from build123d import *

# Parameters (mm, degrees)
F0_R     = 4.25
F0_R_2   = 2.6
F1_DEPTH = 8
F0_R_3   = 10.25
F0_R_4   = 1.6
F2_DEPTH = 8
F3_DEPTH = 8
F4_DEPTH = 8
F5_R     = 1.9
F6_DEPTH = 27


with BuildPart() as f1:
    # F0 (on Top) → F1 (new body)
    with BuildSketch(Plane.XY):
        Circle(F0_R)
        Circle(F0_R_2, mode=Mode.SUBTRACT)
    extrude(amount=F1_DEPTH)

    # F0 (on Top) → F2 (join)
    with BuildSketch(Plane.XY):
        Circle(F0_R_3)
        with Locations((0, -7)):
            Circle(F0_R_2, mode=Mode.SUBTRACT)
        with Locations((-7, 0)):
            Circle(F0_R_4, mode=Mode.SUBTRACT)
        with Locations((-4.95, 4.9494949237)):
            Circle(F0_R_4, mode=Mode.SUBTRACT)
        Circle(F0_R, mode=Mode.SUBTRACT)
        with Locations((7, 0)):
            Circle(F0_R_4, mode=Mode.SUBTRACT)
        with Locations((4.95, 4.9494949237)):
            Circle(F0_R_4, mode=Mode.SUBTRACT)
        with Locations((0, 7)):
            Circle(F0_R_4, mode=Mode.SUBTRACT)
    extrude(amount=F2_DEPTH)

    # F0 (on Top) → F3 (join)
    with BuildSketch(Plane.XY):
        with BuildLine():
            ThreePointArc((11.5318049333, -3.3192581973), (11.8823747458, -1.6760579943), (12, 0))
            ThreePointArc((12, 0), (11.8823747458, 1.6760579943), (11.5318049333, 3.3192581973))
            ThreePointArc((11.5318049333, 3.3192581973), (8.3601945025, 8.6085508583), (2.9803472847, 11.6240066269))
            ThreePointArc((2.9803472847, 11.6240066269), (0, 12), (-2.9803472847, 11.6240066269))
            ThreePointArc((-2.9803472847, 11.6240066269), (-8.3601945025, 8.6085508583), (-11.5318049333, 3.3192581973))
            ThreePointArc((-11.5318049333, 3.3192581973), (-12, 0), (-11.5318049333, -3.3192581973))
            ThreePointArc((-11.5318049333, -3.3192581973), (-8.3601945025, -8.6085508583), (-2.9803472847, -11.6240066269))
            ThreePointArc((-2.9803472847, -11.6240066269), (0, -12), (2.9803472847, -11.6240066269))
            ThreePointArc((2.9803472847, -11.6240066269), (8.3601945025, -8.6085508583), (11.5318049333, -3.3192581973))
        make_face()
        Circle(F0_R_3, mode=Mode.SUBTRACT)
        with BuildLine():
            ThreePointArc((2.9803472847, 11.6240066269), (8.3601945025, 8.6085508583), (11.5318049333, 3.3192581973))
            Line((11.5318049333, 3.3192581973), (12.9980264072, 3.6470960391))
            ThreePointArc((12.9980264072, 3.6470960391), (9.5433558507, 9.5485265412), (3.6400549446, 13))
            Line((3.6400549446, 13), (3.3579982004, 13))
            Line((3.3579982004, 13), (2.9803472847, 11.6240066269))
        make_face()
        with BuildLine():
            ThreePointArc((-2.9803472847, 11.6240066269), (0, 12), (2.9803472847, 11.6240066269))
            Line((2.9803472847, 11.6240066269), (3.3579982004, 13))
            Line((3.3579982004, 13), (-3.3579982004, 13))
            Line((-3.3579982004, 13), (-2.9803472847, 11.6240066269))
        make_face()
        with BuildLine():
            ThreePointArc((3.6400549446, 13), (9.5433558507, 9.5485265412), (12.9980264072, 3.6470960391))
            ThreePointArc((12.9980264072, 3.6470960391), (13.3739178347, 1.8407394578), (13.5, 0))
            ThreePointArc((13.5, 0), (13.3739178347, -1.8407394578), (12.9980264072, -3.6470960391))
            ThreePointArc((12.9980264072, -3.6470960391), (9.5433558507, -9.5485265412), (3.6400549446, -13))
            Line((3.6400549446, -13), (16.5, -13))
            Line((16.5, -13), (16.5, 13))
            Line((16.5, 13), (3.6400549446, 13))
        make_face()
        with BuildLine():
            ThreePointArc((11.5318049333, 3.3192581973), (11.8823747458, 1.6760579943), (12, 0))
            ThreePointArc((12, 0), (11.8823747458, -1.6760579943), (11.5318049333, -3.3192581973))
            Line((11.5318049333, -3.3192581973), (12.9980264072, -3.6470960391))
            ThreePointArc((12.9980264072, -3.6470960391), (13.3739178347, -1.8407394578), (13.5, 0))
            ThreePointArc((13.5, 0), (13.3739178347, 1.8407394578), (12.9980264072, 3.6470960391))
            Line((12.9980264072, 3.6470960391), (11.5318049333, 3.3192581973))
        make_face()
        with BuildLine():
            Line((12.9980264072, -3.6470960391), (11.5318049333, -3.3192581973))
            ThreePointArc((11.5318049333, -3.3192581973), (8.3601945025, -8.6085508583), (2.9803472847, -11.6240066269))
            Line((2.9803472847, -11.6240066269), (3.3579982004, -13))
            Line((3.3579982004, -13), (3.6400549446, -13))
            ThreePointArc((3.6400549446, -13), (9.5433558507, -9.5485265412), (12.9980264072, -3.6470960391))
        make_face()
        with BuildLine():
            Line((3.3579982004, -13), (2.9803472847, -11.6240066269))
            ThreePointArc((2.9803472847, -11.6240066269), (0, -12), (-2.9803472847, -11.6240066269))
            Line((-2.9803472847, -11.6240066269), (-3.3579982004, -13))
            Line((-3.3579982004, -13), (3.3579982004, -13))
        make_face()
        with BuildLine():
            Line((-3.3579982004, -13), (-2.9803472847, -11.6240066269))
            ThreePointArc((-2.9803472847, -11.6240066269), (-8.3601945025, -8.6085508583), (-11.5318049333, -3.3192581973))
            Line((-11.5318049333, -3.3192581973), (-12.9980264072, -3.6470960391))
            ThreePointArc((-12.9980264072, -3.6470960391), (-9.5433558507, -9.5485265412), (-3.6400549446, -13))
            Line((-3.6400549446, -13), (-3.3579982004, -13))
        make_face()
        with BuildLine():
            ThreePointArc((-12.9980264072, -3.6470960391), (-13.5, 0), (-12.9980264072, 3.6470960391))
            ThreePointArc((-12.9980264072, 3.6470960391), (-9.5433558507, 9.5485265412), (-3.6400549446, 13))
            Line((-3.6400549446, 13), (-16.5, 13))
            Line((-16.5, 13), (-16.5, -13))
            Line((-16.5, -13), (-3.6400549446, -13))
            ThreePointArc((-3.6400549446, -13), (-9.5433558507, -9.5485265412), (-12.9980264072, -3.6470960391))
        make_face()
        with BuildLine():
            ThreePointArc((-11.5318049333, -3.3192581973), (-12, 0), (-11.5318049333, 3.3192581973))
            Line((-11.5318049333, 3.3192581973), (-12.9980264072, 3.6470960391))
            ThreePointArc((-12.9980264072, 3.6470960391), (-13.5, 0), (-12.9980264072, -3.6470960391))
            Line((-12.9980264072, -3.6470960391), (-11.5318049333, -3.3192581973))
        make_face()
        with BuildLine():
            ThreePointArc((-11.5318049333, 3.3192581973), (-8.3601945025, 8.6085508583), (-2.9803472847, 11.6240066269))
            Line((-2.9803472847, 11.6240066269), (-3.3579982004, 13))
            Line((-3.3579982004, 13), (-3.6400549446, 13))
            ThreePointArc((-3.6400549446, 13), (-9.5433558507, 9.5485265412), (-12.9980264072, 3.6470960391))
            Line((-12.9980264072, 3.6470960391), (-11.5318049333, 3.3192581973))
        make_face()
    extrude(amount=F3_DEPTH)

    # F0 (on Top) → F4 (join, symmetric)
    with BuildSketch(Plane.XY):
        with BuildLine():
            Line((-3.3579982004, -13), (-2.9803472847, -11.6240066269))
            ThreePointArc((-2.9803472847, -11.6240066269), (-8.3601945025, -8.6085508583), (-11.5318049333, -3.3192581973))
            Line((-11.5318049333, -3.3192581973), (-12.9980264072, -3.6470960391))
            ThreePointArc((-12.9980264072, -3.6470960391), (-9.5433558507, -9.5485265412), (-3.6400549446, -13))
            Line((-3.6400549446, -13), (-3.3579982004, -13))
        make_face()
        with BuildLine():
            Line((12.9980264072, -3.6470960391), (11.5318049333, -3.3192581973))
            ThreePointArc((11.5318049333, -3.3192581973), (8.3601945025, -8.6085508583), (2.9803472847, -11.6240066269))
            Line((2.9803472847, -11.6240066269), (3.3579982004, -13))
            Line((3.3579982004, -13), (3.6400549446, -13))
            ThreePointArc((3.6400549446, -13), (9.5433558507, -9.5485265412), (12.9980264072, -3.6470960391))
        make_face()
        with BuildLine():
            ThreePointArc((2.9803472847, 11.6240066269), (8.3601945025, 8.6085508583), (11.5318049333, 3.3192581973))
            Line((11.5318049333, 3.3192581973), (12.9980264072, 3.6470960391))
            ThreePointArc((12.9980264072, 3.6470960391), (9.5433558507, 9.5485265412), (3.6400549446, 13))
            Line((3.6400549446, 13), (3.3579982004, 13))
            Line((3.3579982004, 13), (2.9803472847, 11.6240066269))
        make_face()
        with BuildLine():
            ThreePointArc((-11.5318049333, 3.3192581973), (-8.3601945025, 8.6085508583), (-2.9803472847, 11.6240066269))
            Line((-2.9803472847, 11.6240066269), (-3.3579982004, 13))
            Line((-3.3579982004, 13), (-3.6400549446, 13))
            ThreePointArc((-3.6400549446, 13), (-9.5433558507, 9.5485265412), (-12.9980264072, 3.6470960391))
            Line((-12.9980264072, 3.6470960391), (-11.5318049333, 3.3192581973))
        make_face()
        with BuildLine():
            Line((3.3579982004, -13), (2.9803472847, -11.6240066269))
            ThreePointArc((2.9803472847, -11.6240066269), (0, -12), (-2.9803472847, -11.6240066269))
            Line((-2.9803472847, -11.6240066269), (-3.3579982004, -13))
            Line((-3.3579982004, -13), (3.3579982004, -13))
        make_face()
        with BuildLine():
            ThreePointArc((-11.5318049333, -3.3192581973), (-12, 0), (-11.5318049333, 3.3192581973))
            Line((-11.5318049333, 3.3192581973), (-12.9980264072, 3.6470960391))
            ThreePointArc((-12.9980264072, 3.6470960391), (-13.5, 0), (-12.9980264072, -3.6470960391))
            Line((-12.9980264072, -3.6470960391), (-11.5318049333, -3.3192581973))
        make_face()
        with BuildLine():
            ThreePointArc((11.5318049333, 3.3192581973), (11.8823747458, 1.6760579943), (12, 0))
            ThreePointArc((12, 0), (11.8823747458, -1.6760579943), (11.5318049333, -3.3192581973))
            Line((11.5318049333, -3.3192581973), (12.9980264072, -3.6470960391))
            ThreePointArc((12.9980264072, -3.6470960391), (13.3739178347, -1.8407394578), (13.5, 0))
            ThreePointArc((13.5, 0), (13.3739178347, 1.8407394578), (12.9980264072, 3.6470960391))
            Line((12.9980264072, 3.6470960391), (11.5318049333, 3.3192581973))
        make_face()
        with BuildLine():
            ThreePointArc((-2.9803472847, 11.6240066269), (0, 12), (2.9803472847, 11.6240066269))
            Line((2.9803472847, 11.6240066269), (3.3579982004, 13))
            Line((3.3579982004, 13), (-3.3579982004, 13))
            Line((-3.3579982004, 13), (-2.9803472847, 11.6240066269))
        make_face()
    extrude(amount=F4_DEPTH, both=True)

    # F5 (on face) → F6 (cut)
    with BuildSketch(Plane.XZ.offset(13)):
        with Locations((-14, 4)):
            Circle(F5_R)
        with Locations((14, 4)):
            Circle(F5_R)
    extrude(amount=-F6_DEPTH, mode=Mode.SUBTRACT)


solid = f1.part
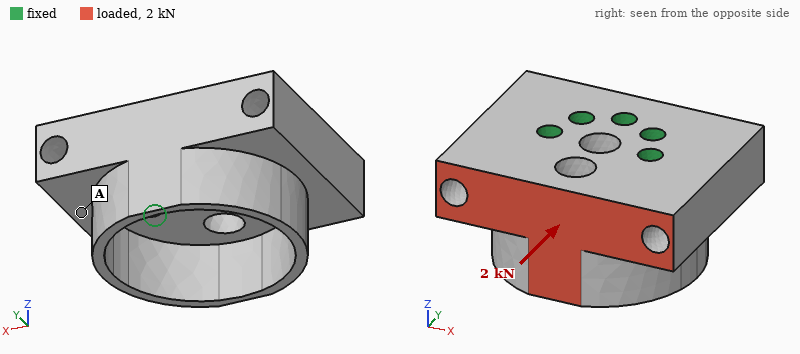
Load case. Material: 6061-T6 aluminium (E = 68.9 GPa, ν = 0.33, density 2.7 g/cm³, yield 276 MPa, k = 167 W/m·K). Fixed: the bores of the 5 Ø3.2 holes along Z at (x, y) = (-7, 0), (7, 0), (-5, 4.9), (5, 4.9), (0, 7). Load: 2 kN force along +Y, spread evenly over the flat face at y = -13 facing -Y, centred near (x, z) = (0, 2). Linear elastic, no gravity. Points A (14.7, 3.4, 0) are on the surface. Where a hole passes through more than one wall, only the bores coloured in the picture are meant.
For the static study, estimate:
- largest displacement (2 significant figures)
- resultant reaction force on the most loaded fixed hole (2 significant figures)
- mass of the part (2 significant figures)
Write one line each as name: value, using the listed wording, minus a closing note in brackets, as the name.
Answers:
largest displacement: 47 µm
resultant reaction force on the most loaded fixed hole: 870 N
mass of the part: 18 g
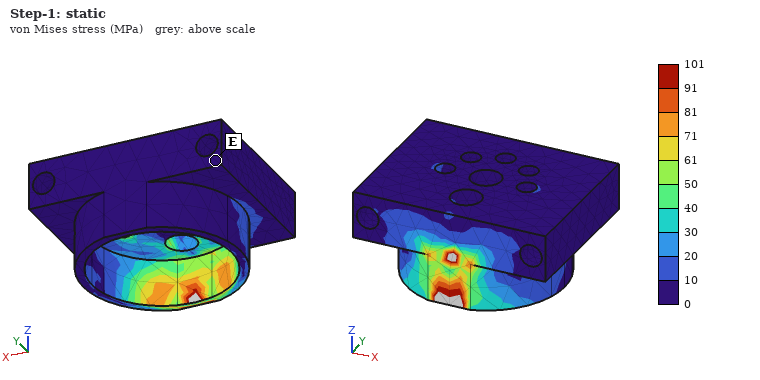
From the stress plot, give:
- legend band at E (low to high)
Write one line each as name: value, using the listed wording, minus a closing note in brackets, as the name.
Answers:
legend band at E: 0 to 10 MPa
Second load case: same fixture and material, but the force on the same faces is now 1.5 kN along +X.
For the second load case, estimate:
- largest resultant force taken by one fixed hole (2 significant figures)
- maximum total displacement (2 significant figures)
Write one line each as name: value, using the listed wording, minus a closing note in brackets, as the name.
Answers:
largest resultant force taken by one fixed hole: 1.3 kN
maximum total displacement: 13 µm
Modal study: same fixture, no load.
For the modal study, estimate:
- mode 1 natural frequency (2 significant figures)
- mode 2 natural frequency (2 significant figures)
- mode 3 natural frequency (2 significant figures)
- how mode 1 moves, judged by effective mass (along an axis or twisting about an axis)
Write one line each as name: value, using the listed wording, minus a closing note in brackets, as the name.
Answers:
mode 1 natural frequency: 24 kHz
mode 2 natural frequency: 25 kHz
mode 3 natural frequency: 30 kHz
how mode 1 moves, judged by effective mass: along Z
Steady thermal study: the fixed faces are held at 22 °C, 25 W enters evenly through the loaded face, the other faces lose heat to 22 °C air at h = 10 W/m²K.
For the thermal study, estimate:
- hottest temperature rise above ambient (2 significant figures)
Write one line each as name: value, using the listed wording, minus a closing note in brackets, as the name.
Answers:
hottest temperature rise above ambient: 15 K
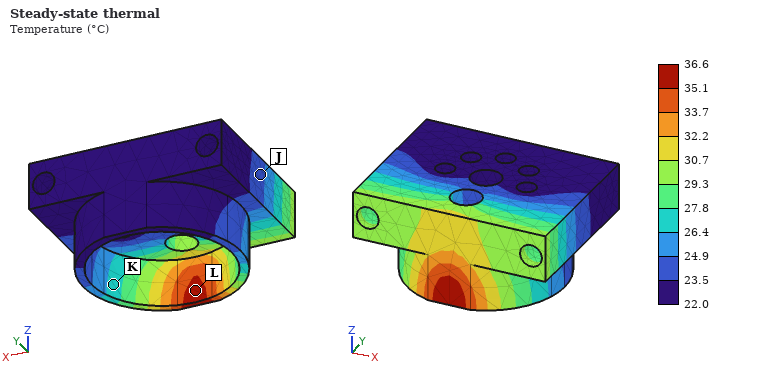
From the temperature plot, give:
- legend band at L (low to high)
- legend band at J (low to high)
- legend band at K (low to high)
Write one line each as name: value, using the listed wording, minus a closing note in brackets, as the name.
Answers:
legend band at L: 35.1 to 36.6 °C
legend band at J: 23.5 to 24.9 °C
legend band at K: 26.4 to 27.8 °C
